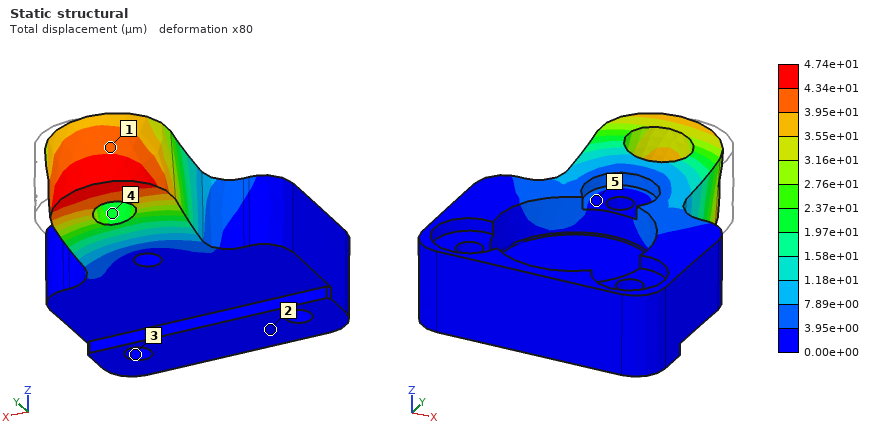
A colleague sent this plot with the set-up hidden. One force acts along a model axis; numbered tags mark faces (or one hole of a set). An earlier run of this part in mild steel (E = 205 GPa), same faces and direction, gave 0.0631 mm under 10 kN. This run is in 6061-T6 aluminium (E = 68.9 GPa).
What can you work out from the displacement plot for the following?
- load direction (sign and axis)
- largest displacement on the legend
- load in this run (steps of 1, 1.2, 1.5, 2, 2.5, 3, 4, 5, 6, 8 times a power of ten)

-X
4.74e+01 µm
2.5 kN
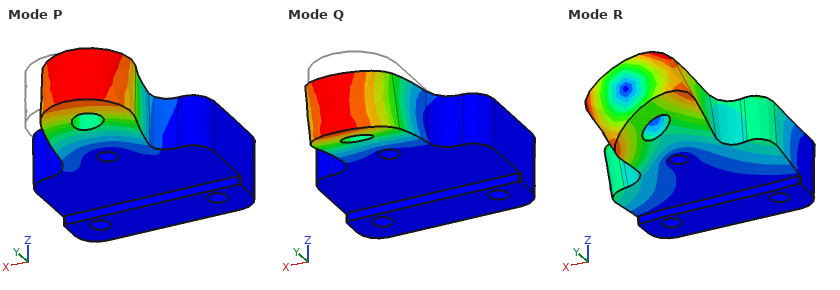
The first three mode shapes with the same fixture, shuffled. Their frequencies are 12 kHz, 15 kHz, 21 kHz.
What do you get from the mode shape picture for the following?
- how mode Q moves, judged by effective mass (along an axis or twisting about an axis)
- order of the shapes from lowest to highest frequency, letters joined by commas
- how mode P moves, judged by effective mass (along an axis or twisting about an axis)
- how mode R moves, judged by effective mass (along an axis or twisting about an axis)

along Z
Q, P, R
along X
twisting about Y
